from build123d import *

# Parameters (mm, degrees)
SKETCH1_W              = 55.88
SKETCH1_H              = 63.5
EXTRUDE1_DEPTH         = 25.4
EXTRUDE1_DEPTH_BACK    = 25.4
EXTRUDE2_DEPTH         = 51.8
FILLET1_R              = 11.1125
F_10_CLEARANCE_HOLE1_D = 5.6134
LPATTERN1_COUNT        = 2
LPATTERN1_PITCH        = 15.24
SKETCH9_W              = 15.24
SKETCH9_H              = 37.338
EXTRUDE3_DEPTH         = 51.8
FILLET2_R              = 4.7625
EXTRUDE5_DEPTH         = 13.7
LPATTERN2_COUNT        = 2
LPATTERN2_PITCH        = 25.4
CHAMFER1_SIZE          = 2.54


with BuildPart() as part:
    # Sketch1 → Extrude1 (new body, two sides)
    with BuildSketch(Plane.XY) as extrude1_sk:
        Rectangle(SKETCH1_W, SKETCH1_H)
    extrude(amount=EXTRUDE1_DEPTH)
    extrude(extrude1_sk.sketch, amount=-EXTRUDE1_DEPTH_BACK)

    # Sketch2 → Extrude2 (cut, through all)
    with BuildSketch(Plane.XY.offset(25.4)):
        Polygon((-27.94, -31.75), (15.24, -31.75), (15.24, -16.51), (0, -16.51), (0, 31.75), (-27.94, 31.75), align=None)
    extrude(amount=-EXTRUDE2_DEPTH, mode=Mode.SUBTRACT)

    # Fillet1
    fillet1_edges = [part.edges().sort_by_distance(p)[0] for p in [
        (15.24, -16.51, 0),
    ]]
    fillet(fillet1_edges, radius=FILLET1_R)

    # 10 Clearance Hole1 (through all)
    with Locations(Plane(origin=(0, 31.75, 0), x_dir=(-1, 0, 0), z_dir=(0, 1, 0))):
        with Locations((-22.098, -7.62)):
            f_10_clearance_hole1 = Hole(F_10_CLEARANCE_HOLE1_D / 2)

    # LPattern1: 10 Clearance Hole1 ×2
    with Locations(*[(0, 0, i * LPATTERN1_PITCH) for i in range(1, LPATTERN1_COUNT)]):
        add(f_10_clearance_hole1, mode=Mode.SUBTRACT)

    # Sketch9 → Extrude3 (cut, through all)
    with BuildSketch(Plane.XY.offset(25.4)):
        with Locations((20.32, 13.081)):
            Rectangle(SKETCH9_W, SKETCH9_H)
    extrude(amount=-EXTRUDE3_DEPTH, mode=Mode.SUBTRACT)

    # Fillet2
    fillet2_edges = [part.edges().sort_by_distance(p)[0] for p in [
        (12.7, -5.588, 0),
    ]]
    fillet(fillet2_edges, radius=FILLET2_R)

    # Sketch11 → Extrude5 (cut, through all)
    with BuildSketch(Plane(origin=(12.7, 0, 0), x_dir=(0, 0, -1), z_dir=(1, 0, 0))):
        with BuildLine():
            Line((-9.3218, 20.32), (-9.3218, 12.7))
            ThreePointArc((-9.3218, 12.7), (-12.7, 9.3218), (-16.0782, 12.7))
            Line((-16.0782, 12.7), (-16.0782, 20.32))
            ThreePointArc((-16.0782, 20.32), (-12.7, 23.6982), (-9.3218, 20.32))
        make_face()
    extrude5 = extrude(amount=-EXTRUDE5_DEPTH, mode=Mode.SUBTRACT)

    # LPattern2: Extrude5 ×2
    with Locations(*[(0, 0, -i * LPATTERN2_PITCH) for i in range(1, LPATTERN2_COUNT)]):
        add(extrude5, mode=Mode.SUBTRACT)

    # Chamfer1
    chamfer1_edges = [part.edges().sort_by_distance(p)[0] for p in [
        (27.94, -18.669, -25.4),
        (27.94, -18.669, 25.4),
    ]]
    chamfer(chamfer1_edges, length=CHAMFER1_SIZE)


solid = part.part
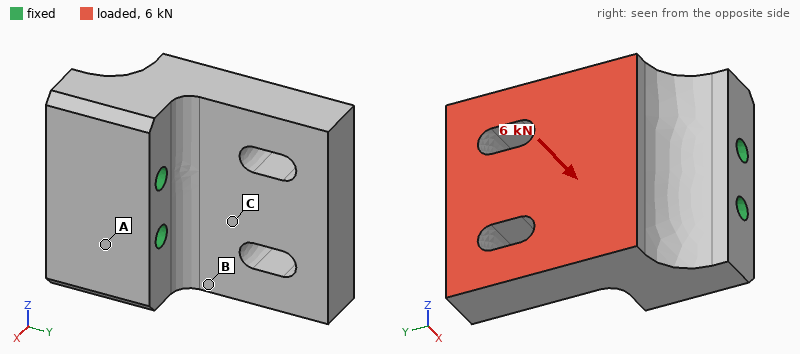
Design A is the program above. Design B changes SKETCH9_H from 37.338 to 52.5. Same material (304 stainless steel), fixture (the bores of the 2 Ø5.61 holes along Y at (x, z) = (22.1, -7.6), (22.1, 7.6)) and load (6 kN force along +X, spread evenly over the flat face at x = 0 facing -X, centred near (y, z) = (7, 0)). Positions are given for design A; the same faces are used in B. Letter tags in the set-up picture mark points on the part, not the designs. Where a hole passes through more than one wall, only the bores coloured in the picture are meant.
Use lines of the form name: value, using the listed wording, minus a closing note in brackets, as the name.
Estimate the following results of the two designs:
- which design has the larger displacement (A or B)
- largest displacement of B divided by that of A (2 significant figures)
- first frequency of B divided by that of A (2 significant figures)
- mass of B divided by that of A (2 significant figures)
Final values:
which design has the larger displacement: B
largest displacement of B divided by that of A: 4.1
first frequency of B divided by that of A: 0.49
mass of B divided by that of A: 0.88
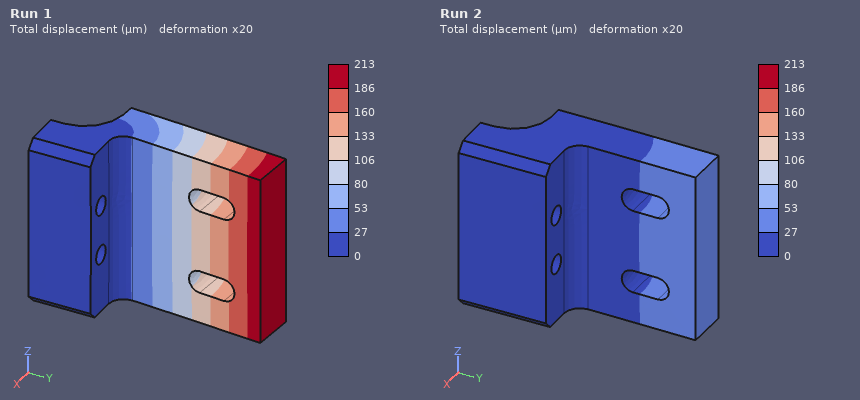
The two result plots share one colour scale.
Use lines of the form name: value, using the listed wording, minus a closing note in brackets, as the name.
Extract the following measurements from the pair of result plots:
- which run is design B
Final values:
which run is design B: Run 1
